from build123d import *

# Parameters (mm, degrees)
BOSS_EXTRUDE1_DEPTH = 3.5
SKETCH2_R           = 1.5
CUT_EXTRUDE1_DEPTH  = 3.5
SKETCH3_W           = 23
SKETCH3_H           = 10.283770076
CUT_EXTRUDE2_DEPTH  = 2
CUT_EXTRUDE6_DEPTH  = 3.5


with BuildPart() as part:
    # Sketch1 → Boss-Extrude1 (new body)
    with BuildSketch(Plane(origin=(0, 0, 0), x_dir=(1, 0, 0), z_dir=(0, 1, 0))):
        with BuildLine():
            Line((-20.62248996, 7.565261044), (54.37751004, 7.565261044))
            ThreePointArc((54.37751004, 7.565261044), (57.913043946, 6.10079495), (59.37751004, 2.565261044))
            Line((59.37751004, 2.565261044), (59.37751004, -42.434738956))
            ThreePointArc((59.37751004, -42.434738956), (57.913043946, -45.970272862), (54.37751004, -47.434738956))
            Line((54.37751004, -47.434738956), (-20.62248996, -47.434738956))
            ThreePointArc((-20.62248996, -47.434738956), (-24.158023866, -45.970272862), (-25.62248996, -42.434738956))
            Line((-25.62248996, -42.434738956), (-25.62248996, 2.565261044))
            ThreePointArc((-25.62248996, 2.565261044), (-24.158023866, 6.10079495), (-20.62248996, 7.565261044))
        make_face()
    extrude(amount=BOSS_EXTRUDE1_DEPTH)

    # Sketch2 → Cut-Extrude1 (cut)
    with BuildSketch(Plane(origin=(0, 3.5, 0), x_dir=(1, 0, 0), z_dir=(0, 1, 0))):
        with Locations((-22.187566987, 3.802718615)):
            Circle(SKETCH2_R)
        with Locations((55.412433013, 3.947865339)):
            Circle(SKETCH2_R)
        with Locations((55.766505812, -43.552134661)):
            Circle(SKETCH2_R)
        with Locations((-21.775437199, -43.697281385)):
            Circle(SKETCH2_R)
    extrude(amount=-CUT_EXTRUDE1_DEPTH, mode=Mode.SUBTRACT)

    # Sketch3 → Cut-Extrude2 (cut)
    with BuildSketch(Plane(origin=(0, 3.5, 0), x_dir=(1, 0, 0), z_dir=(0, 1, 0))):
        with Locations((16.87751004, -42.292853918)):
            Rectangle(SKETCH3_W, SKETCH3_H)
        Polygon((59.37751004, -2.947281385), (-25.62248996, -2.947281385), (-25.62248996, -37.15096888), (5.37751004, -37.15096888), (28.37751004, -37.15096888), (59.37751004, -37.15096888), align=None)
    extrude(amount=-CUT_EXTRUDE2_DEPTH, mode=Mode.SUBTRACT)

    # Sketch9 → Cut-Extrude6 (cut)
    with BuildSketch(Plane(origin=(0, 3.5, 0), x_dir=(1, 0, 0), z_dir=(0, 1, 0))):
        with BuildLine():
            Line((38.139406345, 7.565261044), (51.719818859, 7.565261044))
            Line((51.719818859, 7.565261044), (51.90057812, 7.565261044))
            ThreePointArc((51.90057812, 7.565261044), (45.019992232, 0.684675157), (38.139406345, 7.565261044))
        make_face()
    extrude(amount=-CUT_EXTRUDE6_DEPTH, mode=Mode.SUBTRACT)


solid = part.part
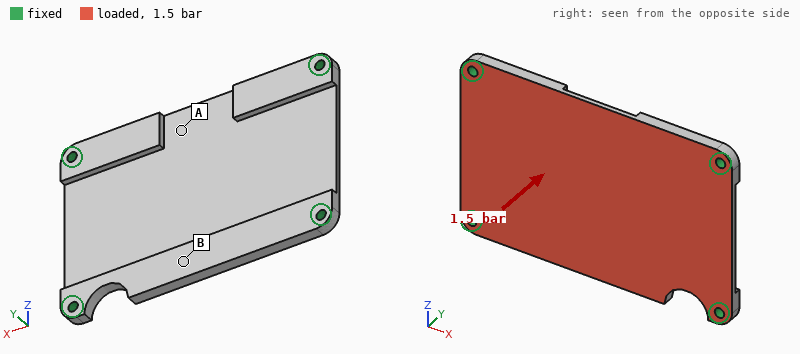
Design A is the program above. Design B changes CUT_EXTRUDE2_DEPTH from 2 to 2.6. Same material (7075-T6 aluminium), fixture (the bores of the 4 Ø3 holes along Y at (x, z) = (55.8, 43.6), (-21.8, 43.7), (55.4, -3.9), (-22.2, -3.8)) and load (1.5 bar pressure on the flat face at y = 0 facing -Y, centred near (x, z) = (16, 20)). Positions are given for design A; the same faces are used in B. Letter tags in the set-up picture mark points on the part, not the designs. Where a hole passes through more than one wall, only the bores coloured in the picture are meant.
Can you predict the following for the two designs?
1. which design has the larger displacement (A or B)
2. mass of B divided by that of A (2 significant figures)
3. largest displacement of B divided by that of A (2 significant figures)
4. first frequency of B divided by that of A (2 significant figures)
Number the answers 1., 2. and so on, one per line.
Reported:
1. B
2. 0.80
3. 1.6
4. 1.0
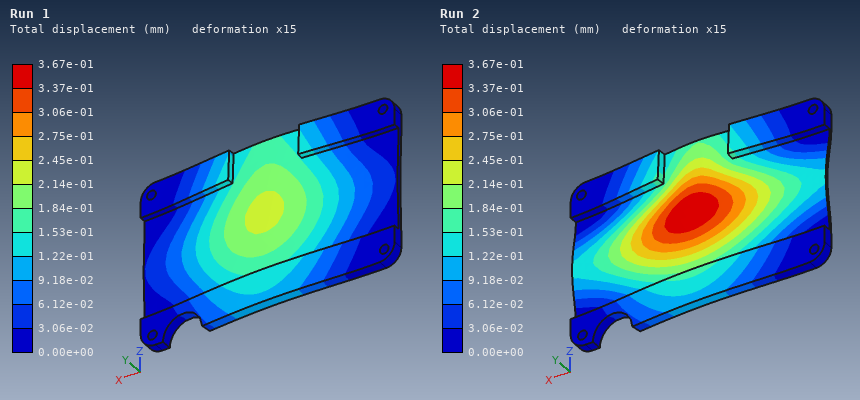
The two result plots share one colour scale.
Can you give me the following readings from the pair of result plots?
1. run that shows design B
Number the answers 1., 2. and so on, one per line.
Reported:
1. Run 2
